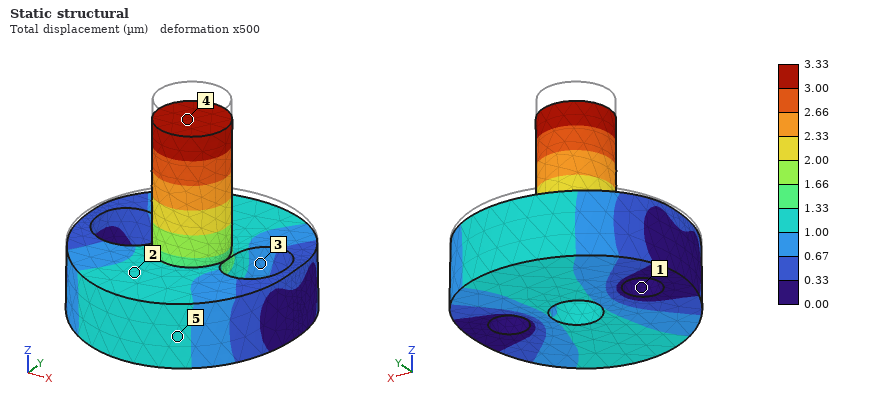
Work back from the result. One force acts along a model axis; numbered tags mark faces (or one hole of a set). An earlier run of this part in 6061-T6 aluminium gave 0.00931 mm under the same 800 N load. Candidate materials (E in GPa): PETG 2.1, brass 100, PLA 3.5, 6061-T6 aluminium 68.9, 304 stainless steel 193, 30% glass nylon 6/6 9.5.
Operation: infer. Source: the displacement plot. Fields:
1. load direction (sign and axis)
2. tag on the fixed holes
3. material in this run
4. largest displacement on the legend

-Z
1
304 stainless steel
3.33 µm
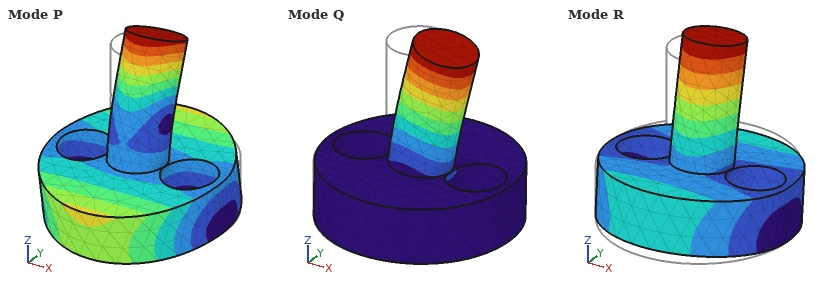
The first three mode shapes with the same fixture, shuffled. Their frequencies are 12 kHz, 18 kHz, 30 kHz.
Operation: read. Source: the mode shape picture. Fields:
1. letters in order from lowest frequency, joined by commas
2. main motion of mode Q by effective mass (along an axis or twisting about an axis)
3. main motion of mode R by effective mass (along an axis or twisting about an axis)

R, Q, P
along X
along Y
